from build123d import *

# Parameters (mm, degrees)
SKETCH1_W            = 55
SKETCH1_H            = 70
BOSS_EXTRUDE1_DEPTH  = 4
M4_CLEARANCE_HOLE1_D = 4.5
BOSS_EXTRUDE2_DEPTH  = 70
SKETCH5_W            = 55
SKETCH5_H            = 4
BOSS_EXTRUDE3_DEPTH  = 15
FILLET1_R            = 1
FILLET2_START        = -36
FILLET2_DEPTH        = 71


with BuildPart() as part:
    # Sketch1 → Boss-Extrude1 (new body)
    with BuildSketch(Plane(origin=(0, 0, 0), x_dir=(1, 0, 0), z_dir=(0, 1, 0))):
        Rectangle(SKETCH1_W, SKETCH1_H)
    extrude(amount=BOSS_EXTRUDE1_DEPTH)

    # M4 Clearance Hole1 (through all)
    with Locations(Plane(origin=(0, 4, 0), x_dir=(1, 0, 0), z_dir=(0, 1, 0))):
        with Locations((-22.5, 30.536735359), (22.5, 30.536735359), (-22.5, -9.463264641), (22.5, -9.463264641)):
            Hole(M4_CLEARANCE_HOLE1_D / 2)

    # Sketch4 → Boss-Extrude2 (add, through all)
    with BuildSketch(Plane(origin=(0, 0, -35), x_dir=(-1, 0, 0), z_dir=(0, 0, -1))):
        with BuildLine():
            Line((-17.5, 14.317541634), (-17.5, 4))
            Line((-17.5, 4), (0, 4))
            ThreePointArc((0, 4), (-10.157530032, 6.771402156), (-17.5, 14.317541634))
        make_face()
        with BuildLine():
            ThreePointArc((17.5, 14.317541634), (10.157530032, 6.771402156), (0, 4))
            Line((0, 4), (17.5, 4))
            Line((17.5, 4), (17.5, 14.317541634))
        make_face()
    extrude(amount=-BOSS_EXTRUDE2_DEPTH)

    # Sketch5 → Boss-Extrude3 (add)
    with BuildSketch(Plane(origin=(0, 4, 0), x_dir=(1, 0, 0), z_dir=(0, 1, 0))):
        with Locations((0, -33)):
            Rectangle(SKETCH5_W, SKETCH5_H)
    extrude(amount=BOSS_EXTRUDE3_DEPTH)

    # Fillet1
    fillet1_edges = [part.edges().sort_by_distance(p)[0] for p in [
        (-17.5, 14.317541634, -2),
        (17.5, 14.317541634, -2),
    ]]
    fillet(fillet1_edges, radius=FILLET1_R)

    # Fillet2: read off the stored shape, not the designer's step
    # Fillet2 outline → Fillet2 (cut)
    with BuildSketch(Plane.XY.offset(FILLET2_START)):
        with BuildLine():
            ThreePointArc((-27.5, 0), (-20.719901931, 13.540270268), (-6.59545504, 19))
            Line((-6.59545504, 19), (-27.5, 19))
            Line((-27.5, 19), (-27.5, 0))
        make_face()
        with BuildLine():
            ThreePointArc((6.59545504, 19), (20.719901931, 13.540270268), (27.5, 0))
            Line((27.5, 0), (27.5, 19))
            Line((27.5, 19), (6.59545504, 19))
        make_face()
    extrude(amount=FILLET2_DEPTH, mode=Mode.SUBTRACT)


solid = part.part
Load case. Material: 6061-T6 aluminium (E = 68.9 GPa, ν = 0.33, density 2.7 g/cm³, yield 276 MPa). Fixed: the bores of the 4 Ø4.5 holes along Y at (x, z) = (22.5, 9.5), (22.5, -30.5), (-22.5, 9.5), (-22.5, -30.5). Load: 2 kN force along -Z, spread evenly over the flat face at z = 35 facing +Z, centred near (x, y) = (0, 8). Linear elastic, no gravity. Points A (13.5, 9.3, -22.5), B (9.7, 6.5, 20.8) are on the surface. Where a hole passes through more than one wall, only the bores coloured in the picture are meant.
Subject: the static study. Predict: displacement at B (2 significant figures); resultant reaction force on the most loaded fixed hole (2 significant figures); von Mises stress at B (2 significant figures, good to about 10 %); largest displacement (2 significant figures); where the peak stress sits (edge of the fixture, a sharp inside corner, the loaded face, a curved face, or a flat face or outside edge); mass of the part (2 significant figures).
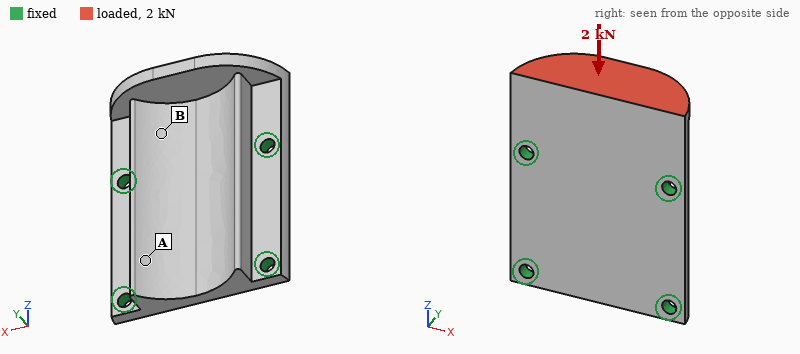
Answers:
16 µm
620 N
21 MPa
81 µm
a curved face
65 g
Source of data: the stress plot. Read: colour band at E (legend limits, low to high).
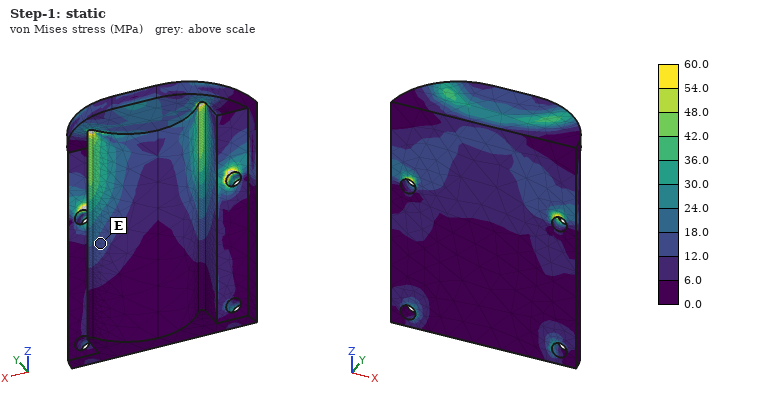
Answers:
12.0 to 18.0 MPa
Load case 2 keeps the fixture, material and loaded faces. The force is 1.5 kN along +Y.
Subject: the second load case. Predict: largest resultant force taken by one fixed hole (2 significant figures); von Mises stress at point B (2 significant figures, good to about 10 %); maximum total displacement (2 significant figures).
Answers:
1.4 kN
34 MPa
0.17 mm
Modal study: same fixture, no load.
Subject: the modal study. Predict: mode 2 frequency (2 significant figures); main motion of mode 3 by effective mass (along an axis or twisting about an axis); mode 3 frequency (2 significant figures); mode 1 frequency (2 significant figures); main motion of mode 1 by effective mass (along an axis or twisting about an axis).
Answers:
7700 Hz
along Y
8500 Hz
4600 Hz
along Y
